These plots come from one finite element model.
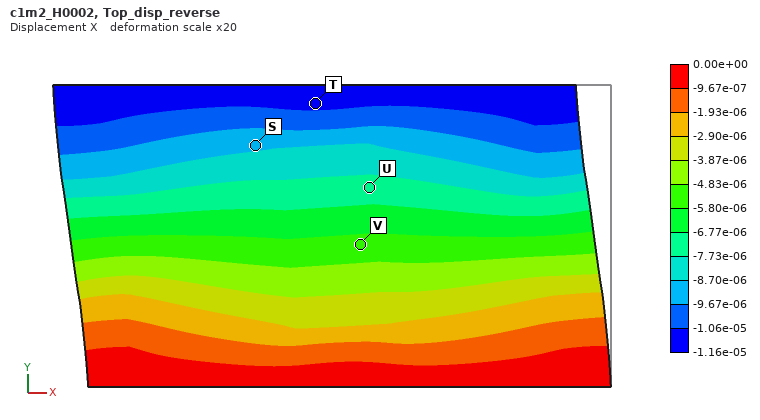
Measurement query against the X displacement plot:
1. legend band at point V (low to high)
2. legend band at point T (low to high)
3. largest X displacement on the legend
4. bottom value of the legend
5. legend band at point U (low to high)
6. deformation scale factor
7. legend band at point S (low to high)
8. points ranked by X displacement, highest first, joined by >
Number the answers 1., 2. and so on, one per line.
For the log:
1. -5.80e-06 to -4.83e-06
2. -1.16e-05 to -1.06e-05
3. 0.00e+00
4. -1.16e-05
5. -7.73e-06 to -6.77e-06
6. 20
7. -9.67e-06 to -8.70e-06
8. V > U > S > T
